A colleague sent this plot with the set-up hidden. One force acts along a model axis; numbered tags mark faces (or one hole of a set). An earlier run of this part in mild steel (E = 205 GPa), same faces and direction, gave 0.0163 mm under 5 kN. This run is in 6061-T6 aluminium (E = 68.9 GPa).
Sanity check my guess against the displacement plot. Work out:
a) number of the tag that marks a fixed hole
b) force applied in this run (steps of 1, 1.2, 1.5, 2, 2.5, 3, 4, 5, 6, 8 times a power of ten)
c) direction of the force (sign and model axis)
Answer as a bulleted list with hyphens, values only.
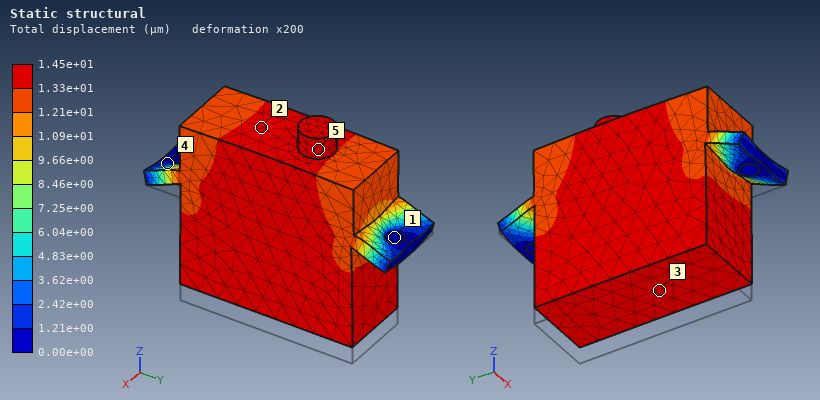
- 1
- 1.5 kN
- +Z
